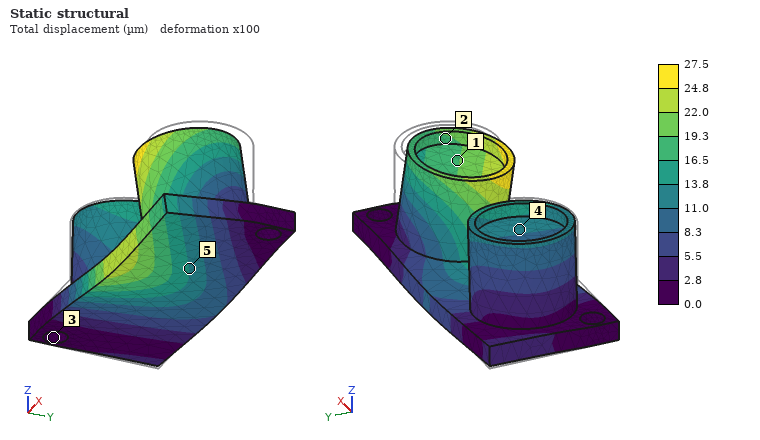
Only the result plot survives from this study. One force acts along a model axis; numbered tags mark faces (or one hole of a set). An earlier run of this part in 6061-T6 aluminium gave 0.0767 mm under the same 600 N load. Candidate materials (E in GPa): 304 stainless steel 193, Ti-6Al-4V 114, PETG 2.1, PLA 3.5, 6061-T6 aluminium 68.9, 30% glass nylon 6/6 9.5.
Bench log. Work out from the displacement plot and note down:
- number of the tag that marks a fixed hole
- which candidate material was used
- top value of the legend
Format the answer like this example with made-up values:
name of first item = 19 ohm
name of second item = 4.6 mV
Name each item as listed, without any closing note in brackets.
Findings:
number of the tag that marks a fixed hole = 3
which candidate material was used = 304 stainless steel
top value of the legend = 27.5 µm
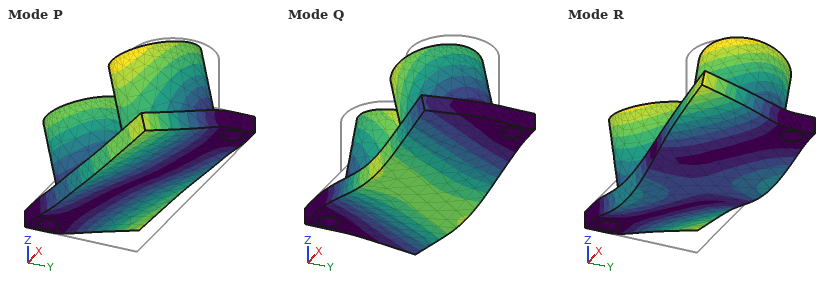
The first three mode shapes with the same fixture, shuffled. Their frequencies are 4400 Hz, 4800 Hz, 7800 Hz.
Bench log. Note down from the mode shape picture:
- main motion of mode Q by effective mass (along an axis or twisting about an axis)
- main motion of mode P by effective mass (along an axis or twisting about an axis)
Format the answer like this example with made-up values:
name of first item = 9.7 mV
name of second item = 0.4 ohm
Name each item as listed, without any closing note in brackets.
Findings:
main motion of mode Q by effective mass = along Z
main motion of mode P by effective mass = along Y
